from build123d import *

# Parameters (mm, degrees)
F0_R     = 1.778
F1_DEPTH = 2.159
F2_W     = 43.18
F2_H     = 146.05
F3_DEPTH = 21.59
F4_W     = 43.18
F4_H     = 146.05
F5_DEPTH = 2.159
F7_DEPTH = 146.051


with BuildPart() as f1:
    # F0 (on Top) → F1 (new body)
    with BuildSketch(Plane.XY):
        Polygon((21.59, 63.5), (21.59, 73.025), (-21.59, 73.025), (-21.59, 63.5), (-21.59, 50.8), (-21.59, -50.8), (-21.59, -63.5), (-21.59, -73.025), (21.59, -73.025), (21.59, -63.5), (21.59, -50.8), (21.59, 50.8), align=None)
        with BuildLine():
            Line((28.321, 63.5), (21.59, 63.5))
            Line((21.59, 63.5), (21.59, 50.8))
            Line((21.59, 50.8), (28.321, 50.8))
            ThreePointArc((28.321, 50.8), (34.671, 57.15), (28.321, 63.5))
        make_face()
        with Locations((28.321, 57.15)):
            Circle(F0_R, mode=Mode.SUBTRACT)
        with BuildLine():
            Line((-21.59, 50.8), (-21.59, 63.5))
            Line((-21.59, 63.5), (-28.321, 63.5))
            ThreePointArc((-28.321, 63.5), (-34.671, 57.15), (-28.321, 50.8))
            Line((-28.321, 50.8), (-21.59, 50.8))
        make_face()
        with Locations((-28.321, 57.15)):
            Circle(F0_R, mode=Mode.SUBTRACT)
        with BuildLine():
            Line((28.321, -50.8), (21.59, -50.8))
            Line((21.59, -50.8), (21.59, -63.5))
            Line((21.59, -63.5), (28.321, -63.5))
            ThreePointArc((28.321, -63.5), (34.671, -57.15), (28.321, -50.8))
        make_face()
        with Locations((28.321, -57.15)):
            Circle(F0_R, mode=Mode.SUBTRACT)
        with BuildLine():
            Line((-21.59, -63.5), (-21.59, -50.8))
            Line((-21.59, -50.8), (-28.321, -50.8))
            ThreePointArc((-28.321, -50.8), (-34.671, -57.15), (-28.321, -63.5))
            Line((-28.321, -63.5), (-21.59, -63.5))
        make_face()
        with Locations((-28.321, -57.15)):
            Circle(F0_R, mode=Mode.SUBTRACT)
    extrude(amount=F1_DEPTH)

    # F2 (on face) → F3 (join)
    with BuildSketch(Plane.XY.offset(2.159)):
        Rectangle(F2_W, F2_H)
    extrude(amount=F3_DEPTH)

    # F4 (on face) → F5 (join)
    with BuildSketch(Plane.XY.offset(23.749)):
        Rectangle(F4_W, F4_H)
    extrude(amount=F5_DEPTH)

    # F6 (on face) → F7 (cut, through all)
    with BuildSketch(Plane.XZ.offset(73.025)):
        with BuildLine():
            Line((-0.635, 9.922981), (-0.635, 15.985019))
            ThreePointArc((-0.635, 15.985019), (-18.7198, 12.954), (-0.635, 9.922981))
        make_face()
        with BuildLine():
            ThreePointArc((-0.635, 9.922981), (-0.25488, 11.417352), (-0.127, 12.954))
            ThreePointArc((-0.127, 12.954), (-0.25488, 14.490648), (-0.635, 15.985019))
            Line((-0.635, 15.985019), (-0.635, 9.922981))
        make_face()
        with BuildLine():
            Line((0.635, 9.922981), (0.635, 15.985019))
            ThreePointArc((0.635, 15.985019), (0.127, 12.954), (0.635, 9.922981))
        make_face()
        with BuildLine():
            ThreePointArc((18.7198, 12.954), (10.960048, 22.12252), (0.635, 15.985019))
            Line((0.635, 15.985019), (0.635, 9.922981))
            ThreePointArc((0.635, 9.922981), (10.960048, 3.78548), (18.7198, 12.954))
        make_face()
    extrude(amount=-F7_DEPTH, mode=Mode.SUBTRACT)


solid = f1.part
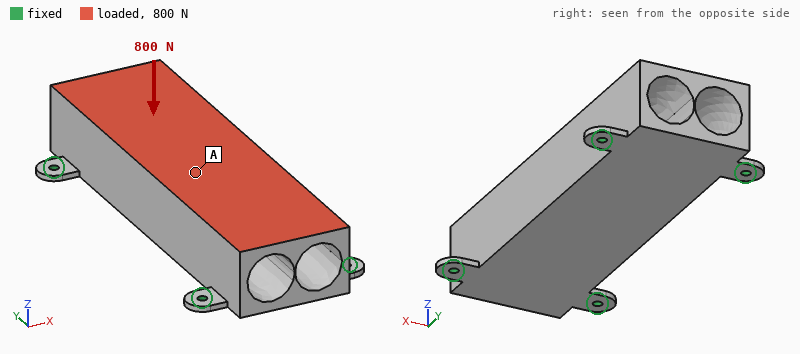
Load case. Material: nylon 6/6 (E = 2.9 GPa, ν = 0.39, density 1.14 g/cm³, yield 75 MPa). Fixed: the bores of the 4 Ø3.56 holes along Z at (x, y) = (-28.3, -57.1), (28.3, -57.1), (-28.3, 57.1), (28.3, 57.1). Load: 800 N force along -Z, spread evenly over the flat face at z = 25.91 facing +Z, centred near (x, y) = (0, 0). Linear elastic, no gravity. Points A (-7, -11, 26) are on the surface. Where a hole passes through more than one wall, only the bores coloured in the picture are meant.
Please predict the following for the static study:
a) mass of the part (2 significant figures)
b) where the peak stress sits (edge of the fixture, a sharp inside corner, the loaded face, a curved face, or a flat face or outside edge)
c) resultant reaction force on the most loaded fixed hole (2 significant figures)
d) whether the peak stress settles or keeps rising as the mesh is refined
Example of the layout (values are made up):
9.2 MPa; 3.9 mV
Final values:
97 g; edge of the fixture; 220 N; keeps rising
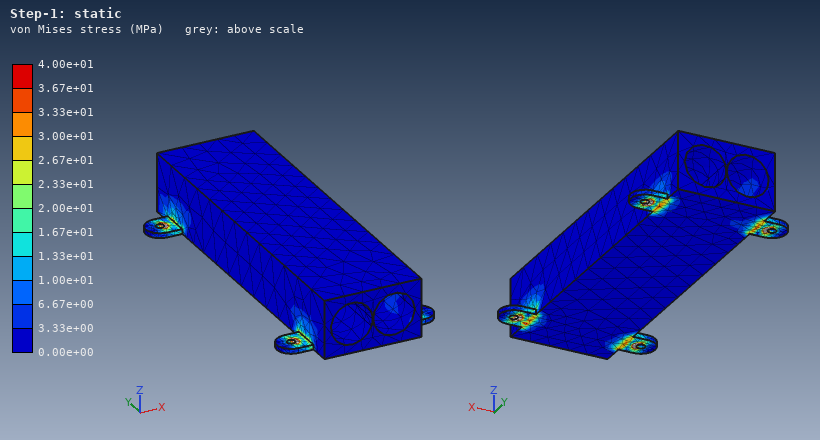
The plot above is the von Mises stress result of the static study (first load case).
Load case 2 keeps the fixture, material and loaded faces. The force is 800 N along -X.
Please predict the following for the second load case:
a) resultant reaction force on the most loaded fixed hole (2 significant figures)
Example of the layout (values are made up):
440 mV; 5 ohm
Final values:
290 N
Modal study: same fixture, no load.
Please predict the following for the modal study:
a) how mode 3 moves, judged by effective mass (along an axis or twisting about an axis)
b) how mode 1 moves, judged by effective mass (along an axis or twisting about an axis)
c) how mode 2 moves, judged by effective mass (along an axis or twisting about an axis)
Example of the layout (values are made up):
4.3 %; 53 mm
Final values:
along Y; along Z; along X
